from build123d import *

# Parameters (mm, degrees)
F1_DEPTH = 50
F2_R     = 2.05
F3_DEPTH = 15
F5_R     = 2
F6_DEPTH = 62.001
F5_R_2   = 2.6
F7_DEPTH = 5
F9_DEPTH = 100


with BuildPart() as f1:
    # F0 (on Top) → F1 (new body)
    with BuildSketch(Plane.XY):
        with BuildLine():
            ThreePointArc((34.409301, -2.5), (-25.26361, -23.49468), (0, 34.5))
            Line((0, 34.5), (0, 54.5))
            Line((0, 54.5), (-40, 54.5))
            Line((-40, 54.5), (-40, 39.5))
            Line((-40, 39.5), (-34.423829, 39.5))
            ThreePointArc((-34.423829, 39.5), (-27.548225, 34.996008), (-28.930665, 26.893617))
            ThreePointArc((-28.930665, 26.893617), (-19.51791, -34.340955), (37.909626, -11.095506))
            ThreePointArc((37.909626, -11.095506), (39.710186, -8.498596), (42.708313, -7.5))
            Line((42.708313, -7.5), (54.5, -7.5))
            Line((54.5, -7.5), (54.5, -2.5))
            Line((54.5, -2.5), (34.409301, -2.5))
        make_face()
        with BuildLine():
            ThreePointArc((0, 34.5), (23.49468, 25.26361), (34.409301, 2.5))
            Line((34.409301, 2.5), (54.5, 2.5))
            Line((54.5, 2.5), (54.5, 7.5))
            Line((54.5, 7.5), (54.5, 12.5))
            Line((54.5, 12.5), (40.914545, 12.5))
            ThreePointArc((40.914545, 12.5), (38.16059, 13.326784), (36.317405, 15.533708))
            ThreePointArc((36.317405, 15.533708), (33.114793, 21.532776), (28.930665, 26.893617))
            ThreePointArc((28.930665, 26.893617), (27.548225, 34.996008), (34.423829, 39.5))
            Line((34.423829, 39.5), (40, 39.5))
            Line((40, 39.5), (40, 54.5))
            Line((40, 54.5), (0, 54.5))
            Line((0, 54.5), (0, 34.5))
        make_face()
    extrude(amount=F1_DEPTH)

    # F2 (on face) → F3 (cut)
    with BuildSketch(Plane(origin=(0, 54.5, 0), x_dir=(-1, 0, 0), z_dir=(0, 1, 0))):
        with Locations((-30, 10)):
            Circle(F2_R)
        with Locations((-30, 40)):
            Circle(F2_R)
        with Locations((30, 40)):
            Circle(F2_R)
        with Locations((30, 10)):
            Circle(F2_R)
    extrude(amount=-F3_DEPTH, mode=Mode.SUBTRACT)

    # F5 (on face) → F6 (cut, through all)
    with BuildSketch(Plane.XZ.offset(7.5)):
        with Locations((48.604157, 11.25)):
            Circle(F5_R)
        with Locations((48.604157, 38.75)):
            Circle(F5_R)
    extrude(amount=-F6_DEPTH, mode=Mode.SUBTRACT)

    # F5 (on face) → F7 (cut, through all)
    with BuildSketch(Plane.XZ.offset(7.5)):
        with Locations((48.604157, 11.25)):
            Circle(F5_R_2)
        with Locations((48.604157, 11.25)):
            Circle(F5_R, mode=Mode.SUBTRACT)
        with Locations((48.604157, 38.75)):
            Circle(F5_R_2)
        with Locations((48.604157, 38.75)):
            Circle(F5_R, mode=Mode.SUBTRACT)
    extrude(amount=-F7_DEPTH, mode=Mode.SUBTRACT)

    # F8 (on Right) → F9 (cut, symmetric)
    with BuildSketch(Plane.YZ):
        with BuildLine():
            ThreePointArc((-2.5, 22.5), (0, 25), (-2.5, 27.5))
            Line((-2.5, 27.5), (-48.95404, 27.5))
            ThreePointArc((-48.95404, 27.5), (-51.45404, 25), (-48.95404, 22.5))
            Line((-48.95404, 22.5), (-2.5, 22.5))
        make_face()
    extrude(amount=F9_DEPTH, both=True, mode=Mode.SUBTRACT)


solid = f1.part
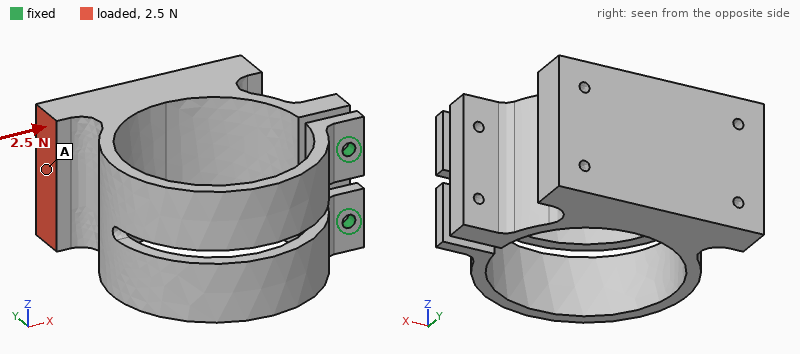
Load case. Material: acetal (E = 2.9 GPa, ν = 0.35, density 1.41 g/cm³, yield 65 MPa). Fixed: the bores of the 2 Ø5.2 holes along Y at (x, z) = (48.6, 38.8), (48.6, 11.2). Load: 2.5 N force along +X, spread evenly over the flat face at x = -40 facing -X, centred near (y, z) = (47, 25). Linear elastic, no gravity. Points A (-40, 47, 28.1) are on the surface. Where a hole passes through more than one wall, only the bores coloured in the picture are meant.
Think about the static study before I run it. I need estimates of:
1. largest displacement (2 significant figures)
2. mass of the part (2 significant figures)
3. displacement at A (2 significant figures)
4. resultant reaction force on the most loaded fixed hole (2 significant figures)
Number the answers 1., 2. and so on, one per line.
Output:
1. 1.4 mm
2. 190 g
3. 1.3 mm
4. 1.3 N
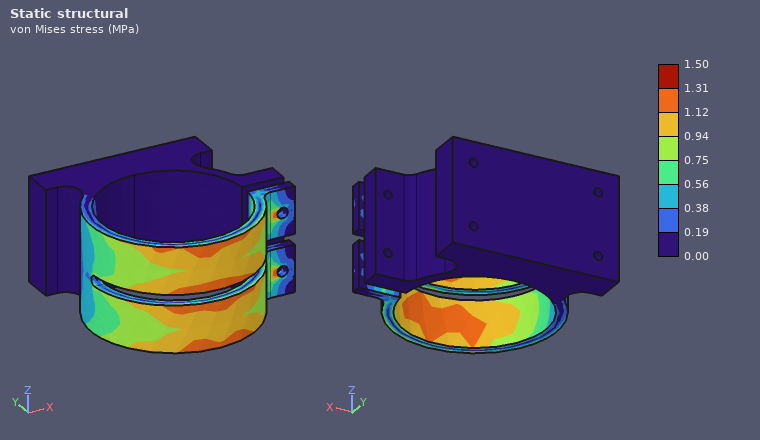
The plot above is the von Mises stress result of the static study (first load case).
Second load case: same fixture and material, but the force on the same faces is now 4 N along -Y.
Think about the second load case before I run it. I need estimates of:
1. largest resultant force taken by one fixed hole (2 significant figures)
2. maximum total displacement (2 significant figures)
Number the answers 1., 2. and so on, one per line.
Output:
1. 2.0 N
2. 1.4 mm
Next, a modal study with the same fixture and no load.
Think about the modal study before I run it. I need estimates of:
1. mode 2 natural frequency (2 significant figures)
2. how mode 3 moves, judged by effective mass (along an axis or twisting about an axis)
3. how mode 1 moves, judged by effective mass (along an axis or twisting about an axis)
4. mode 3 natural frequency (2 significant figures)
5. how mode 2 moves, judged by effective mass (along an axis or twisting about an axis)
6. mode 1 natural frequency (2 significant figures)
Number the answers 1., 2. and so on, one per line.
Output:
1. 26 Hz
2. along Y
3. along X
4. 42 Hz
5. along Z
6. 20 Hz
